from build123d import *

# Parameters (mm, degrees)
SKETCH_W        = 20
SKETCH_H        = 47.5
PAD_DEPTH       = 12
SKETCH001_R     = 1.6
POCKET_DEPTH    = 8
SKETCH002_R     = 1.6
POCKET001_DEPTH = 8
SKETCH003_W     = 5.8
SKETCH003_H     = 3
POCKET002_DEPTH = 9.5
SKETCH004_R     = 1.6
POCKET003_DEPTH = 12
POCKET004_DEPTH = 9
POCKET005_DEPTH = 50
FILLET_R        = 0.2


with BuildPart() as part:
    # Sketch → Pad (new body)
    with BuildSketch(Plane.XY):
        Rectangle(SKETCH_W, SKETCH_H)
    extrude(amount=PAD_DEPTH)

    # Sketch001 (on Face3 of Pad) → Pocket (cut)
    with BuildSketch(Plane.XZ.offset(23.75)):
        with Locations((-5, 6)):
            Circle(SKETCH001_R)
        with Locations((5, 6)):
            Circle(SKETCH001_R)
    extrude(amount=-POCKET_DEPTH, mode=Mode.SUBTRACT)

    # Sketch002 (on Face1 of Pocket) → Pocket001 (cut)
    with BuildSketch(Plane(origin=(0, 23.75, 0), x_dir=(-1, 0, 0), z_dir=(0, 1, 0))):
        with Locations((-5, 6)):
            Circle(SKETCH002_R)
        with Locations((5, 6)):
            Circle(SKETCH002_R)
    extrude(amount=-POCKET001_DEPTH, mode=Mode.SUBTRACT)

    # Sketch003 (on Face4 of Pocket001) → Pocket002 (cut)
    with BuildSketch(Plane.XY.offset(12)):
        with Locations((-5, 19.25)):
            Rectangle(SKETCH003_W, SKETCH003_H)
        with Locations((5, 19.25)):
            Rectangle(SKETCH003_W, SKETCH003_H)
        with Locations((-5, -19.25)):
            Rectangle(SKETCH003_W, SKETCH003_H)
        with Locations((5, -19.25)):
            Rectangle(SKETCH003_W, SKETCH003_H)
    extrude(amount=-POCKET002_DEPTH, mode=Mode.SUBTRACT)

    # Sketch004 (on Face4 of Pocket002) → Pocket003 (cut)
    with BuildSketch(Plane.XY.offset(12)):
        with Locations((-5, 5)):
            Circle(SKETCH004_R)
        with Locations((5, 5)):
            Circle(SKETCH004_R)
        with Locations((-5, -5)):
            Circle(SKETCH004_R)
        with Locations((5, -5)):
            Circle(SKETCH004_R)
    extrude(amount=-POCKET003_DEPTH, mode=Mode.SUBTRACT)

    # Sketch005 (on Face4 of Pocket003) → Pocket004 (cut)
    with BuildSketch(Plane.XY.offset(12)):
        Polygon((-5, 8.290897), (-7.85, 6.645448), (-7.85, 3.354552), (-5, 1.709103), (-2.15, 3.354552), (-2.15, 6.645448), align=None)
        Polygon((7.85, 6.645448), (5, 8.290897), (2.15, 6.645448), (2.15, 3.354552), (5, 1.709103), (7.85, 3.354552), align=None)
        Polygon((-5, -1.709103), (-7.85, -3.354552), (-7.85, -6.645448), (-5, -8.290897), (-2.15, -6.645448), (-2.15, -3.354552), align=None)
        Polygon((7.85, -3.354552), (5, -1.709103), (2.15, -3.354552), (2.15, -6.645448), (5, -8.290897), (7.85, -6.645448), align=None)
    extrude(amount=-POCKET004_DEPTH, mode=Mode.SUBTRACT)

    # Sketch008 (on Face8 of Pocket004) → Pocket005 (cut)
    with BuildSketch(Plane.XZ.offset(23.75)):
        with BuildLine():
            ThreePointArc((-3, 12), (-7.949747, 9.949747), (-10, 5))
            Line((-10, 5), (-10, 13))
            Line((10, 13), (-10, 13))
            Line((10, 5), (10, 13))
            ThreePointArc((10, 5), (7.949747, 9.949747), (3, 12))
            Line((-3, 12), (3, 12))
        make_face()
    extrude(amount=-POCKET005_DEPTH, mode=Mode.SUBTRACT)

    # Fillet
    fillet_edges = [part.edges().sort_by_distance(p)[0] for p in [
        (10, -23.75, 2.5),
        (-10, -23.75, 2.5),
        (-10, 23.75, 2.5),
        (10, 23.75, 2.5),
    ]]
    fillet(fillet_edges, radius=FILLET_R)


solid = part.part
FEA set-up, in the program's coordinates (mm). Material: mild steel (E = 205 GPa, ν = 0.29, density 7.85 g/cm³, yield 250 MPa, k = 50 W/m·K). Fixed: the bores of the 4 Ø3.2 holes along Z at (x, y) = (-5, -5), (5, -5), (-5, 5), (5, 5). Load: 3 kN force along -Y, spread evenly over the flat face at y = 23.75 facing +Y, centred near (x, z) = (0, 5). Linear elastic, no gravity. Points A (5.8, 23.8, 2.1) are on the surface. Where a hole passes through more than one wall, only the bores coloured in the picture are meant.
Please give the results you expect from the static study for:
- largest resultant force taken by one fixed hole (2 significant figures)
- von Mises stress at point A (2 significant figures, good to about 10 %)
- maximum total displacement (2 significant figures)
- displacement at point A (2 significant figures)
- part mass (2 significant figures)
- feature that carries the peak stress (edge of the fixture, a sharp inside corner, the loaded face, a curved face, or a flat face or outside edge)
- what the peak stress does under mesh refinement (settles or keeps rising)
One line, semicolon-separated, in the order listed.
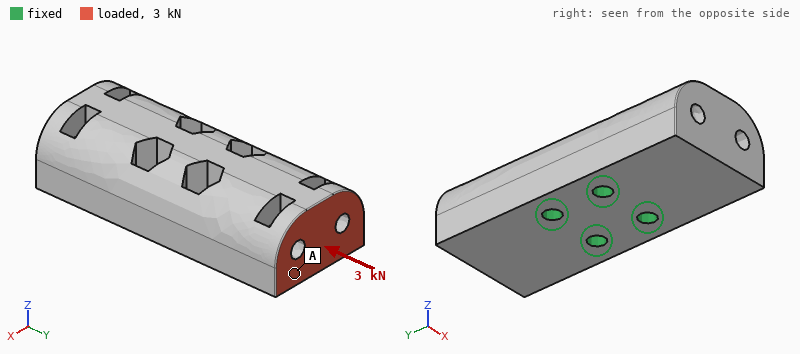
1.1 kN; 14 MPa; 9.0 µm; 6.5 µm; 67 g; edge of the fixture; keeps rising
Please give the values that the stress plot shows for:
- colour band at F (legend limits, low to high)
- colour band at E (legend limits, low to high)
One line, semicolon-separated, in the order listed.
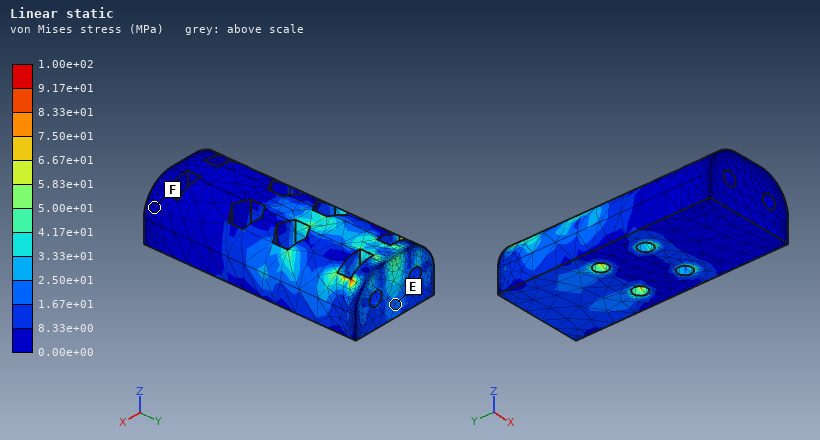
0.00e+00 to 8.33e+00 MPa; 1.67e+01 to 2.50e+01 MPa
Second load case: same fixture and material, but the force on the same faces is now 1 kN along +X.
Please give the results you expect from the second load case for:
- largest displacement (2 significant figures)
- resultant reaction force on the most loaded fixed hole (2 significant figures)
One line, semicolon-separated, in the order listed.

7.0 µm; 1.2 kN
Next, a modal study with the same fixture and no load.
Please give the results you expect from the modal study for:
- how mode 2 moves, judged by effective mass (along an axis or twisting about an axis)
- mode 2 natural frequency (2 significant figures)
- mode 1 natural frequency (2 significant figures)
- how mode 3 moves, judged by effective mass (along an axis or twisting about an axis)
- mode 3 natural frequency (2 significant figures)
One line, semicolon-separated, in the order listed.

along Z; 16 kHz; 11 kHz; twisting about Z; 20 kHz
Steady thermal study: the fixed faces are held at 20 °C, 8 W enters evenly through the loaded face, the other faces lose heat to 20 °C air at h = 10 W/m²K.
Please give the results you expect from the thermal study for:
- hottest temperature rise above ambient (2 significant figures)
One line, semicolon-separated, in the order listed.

23 K
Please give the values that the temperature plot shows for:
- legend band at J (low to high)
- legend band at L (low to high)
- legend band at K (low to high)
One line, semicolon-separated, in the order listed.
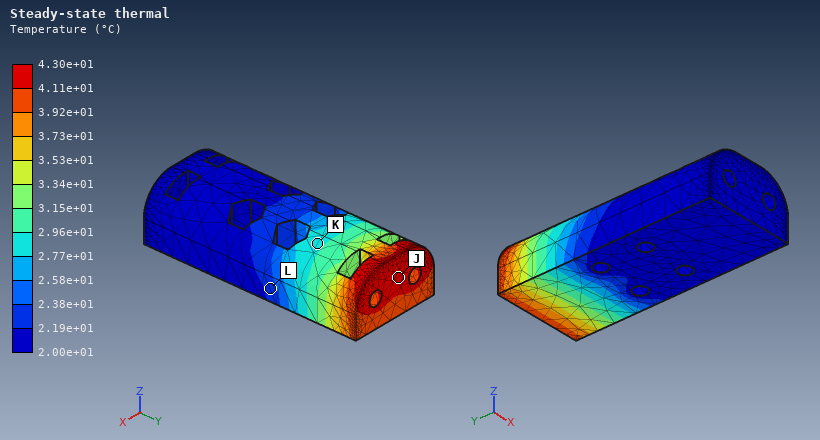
4.11e+01 to 4.30e+01 °C; 2.19e+01 to 2.38e+01 °C; 2.77e+01 to 2.96e+01 °C
